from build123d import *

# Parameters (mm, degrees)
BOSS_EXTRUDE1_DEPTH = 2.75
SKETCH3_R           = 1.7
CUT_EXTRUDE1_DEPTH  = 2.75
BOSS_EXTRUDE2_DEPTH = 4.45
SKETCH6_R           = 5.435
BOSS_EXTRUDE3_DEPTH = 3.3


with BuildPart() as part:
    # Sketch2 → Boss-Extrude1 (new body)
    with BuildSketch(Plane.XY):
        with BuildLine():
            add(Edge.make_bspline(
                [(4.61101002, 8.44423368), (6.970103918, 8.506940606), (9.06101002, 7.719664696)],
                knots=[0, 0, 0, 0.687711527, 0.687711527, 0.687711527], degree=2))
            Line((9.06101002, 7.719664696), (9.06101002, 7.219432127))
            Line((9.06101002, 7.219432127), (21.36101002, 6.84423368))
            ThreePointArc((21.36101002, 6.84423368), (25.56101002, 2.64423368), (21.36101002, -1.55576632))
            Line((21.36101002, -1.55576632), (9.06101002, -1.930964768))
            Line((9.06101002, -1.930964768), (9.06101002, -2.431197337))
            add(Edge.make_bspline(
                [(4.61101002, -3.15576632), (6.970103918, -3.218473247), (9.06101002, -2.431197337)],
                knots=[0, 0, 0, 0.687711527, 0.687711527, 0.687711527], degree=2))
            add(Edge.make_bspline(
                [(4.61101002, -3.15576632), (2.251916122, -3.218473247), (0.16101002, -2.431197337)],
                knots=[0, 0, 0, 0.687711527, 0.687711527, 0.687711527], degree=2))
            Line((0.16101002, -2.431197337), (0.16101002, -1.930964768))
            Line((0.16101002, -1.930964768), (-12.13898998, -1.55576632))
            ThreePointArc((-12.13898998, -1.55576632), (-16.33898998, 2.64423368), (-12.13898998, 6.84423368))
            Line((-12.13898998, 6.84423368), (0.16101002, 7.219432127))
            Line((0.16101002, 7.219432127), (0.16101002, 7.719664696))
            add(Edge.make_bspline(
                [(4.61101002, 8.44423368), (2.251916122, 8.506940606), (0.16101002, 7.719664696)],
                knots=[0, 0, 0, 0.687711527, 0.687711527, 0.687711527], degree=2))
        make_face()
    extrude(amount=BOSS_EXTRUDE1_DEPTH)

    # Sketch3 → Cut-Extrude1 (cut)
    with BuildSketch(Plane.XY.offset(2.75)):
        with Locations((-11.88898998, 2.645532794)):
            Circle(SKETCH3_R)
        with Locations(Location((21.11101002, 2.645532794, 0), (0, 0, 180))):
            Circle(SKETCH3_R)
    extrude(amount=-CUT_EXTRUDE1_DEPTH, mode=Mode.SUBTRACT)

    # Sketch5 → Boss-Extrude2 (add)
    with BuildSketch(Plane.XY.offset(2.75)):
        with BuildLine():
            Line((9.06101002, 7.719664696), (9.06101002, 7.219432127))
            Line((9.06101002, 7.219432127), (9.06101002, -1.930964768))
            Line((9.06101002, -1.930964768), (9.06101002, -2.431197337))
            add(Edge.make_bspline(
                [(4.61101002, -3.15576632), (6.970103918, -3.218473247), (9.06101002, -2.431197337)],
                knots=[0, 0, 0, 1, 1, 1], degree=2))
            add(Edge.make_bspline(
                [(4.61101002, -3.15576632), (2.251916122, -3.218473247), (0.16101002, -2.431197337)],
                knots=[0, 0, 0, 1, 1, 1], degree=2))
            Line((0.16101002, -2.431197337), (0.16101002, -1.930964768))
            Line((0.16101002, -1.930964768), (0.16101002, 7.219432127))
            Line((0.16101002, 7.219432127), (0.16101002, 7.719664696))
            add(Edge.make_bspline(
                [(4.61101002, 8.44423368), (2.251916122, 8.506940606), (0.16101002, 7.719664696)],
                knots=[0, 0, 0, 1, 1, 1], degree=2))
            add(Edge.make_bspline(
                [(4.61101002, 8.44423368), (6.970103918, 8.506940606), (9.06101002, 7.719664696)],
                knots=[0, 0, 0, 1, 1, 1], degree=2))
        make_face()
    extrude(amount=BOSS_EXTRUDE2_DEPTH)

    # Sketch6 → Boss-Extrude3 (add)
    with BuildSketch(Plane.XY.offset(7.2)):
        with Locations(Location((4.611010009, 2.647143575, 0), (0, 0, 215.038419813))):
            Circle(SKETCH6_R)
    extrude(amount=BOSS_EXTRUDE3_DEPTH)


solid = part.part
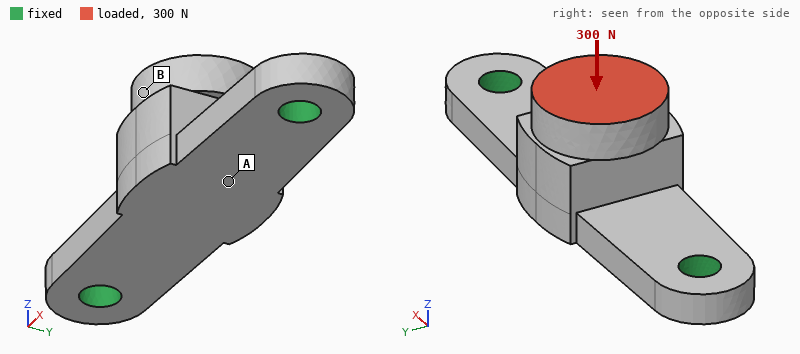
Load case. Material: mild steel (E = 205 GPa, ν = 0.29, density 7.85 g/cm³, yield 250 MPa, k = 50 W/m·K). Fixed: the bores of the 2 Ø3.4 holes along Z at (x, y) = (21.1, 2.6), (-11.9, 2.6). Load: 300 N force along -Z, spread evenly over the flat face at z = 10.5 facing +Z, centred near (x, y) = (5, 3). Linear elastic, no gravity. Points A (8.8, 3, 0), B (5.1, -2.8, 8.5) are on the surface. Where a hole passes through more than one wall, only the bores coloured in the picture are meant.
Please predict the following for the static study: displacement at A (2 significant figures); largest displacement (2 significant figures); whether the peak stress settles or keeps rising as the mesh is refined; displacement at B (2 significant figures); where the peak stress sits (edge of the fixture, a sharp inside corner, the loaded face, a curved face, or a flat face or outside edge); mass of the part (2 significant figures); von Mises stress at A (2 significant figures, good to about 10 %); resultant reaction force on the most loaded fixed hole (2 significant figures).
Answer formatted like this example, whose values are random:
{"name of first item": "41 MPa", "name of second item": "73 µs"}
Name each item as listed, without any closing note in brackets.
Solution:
{"displacement at A": "8.3 µm", "largest displacement": "8.8 µm", "whether the peak stress settles or keeps rising as the mesh is refined": "keeps rising", "displacement at B": "8.7 µm", "where the peak stress sits": "edge of the fixture", "mass of the part": "13 g", "von Mises stress at A": "47 MPa", "resultant reaction force on the most loaded fixed hole": "160 N"}
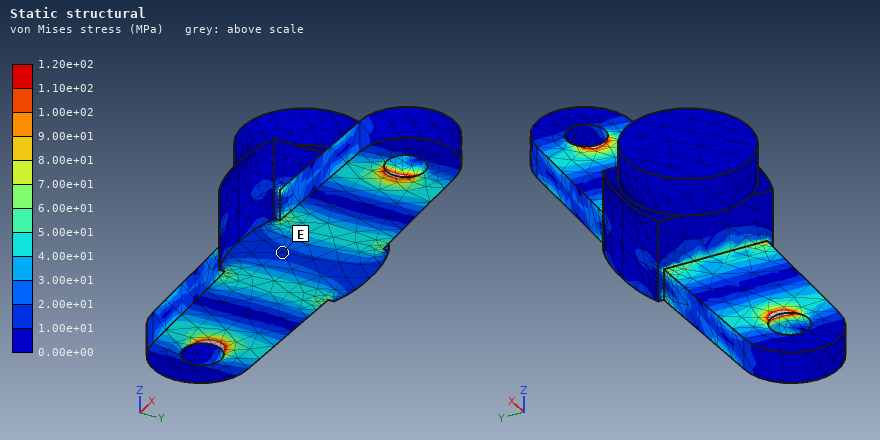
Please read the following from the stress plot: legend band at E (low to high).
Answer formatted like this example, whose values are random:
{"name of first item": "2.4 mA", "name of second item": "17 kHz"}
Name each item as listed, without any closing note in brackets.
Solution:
{"legend band at E": "1.00e+01 to 2.00e+01 MPa"}
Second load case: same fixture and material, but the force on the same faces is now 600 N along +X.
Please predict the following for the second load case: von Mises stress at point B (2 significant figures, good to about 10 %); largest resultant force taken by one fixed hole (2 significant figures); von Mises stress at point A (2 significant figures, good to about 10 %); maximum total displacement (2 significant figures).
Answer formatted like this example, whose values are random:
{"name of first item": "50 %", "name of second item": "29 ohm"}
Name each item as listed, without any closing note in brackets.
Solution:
{"von Mises stress at point B": "17 MPa", "largest resultant force taken by one fixed hole": "390 N", "von Mises stress at point A": "96 MPa", "maximum total displacement": "18 µm"}
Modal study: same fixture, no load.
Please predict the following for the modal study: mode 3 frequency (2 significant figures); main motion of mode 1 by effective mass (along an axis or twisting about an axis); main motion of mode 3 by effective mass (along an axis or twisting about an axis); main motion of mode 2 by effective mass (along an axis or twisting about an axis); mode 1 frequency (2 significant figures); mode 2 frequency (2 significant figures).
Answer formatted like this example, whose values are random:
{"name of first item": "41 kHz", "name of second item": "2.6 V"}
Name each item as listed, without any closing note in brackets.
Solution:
{"mode 3 frequency": "18 kHz", "main motion of mode 1 by effective mass": "along Y", "main motion of mode 3 by effective mass": "along X", "main motion of mode 2 by effective mass": "along Z", "mode 1 frequency": "8000 Hz", "mode 2 frequency": "9700 Hz"}
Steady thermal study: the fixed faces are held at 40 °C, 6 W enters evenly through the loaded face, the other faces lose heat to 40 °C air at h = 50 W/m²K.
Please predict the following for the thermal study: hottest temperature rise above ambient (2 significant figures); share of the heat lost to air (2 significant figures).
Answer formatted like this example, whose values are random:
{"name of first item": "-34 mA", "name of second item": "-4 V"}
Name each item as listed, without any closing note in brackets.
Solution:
{"hottest temperature rise above ambient": "37 K", "share of the heat lost to air": "17 %"}
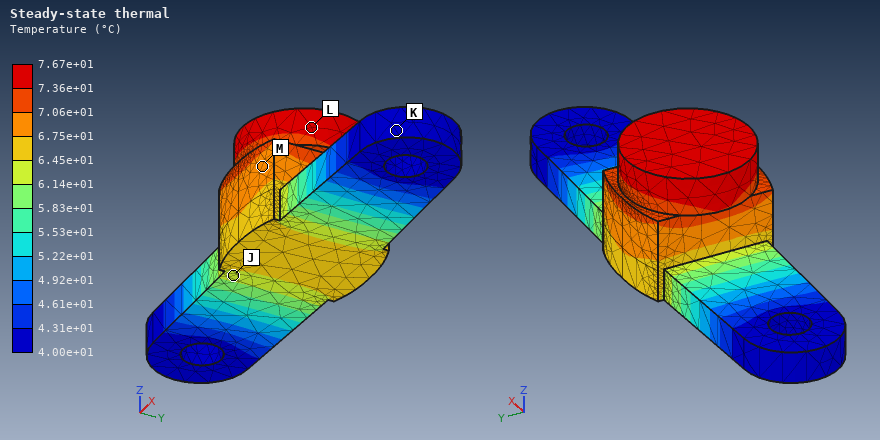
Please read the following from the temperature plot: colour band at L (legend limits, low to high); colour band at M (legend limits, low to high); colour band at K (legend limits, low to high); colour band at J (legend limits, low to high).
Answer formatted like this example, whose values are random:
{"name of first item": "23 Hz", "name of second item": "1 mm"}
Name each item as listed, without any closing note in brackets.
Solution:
{"colour band at L": "7.36e+01 to 7.67e+01 °C", "colour band at M": "6.75e+01 to 7.06e+01 °C", "colour band at K": "4.00e+01 to 4.31e+01 °C", "colour band at J": "6.14e+01 to 6.45e+01 °C"}
